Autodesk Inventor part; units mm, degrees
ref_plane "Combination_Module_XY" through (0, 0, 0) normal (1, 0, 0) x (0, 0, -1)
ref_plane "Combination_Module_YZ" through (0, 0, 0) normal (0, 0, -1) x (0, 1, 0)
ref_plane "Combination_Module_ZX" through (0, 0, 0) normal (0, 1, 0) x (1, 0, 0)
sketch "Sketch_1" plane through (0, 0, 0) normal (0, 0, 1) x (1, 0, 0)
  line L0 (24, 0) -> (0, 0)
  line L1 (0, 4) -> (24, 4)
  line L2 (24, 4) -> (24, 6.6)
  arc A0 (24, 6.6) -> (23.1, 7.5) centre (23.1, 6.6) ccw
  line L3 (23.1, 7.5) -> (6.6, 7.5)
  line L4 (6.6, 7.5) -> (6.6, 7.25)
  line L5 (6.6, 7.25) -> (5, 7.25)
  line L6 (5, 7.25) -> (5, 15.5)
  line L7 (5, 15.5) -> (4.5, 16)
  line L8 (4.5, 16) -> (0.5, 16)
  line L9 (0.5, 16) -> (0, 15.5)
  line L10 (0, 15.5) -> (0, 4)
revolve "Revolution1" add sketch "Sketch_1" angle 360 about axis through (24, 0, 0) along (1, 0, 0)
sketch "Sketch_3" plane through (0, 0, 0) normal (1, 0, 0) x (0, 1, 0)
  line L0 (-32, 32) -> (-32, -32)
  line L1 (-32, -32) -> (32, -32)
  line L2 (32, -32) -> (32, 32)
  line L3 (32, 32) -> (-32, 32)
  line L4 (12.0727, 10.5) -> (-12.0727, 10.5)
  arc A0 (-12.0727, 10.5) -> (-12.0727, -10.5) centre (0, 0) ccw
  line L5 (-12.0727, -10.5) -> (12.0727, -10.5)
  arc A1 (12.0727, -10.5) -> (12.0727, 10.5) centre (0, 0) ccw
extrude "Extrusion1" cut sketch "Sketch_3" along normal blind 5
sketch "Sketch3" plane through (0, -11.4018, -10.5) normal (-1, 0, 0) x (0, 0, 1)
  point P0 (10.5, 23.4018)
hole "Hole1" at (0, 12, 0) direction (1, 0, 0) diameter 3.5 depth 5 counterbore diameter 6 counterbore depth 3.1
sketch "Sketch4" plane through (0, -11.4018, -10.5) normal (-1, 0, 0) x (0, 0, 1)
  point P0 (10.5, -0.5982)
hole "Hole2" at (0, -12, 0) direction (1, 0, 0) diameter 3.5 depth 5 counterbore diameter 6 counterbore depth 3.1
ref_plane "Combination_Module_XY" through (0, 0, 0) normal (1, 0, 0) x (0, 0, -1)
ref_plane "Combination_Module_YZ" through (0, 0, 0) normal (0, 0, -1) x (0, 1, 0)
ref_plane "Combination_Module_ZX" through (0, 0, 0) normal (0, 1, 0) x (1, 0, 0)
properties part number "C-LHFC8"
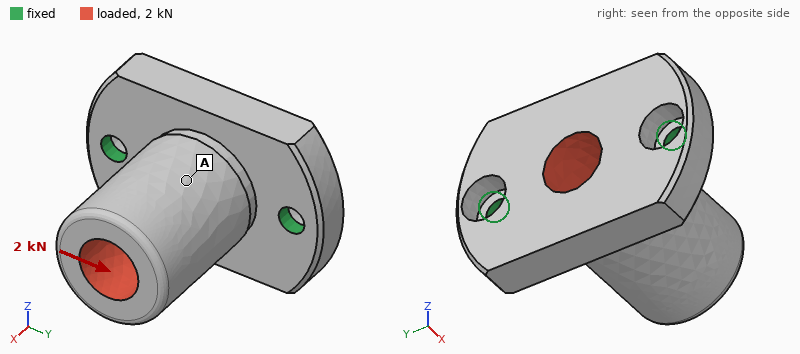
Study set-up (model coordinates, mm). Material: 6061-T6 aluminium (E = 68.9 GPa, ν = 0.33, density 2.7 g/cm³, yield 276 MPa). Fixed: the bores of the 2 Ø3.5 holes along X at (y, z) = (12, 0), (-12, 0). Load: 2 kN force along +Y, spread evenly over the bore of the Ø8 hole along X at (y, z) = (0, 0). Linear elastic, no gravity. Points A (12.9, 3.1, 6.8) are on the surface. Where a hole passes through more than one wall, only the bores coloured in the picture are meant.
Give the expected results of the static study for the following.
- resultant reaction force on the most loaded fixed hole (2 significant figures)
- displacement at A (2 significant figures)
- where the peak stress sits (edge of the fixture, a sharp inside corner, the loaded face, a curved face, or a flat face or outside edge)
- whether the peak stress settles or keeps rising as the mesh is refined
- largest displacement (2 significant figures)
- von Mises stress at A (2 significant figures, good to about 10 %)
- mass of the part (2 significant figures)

1.3 kN
23 µm
edge of the fixture
keeps rising
48 µm
18 MPa
14 g
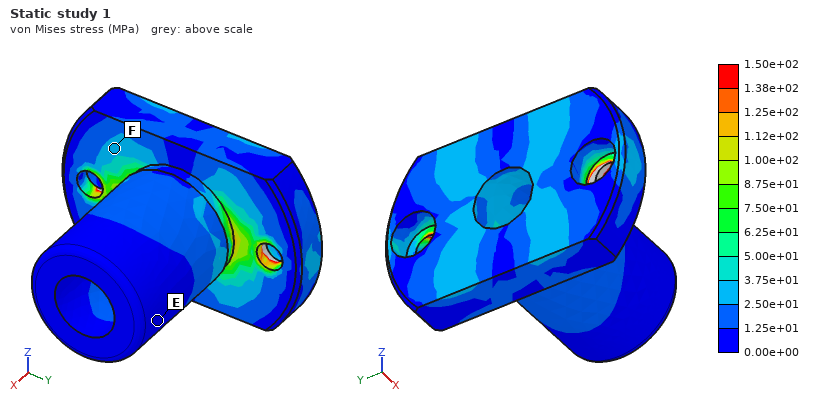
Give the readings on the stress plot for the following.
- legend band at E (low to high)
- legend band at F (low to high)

0.00e+00 to 1.25e+01 MPa
2.50e+01 to 3.75e+01 MPa
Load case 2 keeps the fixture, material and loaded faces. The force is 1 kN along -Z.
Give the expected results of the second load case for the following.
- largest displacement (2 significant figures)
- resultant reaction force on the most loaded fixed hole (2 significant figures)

0.13 mm
500 N
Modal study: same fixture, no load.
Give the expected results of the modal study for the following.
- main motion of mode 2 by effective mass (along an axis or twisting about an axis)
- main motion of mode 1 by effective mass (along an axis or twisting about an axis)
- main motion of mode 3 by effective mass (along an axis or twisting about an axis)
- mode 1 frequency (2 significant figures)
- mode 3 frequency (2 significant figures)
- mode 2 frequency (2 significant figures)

along Y
along Z
along X
5200 Hz
16 kHz
13 kHz
